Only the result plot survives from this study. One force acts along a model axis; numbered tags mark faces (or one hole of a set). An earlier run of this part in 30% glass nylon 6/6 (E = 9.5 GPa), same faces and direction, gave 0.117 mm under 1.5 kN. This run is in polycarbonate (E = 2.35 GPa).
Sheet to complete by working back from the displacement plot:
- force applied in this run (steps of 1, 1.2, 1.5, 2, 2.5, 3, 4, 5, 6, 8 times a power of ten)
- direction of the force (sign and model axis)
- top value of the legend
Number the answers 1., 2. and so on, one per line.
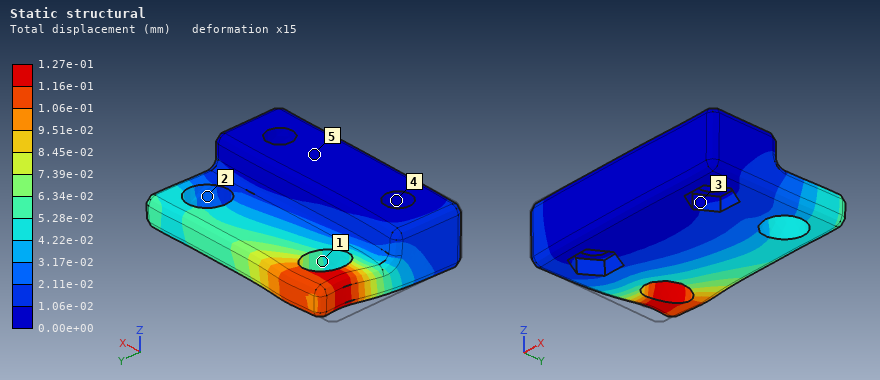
1. 400 N
2. +X
3. 1.27e-01 mm
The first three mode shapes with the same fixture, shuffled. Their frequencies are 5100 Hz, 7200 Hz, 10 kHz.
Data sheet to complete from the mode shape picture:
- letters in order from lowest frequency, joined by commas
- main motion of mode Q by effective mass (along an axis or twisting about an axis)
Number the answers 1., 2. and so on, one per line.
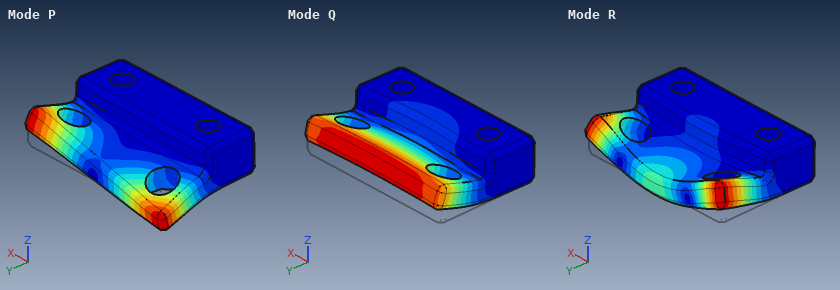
1. Q, P, R
2. along Z
